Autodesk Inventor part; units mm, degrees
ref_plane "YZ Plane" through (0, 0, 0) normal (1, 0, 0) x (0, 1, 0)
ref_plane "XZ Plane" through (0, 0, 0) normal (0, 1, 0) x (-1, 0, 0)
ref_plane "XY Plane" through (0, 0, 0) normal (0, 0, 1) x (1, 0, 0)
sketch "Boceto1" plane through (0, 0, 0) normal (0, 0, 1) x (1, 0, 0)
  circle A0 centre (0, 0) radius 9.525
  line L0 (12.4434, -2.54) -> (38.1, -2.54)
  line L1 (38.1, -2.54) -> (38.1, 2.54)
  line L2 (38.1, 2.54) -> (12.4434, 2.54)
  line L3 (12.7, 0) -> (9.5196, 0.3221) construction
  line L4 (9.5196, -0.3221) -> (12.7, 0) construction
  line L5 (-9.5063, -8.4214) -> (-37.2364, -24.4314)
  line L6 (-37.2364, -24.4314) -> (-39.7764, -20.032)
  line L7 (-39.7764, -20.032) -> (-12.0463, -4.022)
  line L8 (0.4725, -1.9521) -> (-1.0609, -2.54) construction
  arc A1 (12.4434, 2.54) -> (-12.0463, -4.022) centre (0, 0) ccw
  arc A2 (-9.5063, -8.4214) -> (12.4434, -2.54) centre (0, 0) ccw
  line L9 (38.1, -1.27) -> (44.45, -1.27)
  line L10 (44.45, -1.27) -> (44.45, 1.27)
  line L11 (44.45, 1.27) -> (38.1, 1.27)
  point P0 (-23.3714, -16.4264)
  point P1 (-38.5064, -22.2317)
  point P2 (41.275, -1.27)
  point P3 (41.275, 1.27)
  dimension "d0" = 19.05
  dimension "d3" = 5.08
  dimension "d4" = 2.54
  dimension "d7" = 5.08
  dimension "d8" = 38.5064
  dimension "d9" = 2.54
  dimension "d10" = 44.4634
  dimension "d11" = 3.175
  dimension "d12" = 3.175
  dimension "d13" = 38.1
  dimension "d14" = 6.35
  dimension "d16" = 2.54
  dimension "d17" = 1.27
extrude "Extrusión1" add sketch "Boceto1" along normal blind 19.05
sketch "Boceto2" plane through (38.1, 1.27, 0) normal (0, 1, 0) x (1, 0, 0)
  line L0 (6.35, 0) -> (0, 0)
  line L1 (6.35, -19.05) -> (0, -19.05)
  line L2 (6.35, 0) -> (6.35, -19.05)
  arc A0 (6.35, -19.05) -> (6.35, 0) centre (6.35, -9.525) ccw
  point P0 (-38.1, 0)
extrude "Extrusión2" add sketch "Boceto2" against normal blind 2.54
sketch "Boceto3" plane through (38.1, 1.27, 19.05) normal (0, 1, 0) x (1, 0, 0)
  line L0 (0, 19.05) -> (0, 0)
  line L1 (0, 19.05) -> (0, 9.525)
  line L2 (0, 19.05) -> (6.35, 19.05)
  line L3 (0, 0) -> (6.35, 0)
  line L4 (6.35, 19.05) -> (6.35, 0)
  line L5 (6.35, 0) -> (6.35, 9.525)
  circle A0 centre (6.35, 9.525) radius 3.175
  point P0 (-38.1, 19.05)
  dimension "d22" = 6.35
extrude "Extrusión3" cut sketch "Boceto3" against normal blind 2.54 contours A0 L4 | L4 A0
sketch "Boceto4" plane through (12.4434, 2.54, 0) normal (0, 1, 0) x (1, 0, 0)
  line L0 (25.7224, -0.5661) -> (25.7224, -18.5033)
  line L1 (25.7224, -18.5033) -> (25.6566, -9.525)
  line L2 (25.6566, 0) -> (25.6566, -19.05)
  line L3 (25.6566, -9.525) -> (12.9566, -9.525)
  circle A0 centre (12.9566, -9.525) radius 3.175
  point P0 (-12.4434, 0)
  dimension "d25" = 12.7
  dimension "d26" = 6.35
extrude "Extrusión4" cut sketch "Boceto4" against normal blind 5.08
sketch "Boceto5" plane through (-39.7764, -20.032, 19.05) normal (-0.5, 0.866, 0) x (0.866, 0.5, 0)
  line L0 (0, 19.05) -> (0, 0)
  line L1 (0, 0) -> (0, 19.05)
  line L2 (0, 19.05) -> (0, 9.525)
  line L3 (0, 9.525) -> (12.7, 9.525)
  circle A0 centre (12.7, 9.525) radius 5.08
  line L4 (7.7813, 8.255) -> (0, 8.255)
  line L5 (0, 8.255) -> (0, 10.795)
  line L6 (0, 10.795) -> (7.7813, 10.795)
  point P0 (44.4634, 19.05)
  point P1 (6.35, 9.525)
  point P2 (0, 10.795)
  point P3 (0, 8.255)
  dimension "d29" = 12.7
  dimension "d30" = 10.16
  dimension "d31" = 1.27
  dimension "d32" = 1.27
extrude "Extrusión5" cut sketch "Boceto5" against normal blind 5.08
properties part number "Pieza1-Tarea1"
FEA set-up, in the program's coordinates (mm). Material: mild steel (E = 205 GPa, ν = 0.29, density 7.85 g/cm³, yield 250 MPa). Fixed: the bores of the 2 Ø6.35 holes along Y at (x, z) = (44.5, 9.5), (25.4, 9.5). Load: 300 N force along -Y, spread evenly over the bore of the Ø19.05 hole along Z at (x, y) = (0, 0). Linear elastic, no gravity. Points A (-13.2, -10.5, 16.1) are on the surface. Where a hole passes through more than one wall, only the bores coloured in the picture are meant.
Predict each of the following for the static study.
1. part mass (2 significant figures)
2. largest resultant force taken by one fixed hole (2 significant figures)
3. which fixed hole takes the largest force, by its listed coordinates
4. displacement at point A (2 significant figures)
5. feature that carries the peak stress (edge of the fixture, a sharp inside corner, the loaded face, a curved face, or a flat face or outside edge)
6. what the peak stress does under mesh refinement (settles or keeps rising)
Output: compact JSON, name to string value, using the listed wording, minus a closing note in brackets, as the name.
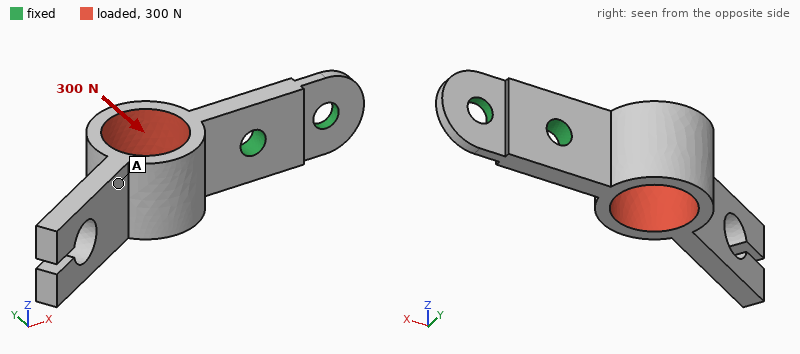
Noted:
{"part mass": "76 g", "largest resultant force taken by one fixed hole": "330 N", "which fixed hole takes the largest force, by its listed coordinates": "(25.4, 9.5)", "displacement at point A": "0.070 mm", "feature that carries the peak stress": "edge of the fixture", "what the peak stress does under mesh refinement": "keeps rising"}
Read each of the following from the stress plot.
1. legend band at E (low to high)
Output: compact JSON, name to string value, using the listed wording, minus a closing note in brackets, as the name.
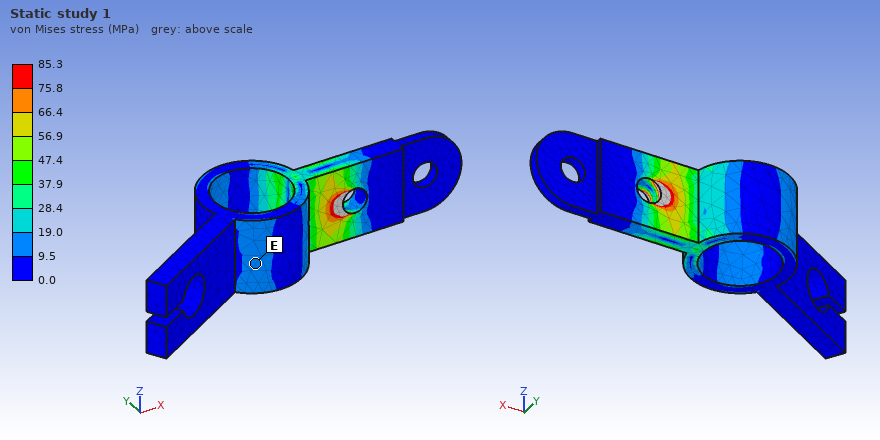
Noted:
{"legend band at E": "9.5 to 19.0 MPa"}
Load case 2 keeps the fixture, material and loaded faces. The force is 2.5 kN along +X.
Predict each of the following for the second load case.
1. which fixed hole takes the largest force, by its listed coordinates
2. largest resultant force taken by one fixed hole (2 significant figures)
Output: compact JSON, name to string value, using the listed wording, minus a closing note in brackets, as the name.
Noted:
{"which fixed hole takes the largest force, by its listed coordinates": "(25.4, 9.5)", "largest resultant force taken by one fixed hole": "2.3 kN"}
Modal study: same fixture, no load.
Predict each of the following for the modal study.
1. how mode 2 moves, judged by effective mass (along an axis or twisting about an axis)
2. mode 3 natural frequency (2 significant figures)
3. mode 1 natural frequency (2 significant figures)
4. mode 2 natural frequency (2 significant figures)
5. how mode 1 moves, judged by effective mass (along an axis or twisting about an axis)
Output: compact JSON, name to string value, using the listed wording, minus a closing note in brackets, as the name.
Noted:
{"how mode 2 moves, judged by effective mass": "along Z", "mode 3 natural frequency": "4900 Hz", "mode 1 natural frequency": "1000 Hz", "mode 2 natural frequency": "1900 Hz", "how mode 1 moves, judged by effective mass": "along Y"}
